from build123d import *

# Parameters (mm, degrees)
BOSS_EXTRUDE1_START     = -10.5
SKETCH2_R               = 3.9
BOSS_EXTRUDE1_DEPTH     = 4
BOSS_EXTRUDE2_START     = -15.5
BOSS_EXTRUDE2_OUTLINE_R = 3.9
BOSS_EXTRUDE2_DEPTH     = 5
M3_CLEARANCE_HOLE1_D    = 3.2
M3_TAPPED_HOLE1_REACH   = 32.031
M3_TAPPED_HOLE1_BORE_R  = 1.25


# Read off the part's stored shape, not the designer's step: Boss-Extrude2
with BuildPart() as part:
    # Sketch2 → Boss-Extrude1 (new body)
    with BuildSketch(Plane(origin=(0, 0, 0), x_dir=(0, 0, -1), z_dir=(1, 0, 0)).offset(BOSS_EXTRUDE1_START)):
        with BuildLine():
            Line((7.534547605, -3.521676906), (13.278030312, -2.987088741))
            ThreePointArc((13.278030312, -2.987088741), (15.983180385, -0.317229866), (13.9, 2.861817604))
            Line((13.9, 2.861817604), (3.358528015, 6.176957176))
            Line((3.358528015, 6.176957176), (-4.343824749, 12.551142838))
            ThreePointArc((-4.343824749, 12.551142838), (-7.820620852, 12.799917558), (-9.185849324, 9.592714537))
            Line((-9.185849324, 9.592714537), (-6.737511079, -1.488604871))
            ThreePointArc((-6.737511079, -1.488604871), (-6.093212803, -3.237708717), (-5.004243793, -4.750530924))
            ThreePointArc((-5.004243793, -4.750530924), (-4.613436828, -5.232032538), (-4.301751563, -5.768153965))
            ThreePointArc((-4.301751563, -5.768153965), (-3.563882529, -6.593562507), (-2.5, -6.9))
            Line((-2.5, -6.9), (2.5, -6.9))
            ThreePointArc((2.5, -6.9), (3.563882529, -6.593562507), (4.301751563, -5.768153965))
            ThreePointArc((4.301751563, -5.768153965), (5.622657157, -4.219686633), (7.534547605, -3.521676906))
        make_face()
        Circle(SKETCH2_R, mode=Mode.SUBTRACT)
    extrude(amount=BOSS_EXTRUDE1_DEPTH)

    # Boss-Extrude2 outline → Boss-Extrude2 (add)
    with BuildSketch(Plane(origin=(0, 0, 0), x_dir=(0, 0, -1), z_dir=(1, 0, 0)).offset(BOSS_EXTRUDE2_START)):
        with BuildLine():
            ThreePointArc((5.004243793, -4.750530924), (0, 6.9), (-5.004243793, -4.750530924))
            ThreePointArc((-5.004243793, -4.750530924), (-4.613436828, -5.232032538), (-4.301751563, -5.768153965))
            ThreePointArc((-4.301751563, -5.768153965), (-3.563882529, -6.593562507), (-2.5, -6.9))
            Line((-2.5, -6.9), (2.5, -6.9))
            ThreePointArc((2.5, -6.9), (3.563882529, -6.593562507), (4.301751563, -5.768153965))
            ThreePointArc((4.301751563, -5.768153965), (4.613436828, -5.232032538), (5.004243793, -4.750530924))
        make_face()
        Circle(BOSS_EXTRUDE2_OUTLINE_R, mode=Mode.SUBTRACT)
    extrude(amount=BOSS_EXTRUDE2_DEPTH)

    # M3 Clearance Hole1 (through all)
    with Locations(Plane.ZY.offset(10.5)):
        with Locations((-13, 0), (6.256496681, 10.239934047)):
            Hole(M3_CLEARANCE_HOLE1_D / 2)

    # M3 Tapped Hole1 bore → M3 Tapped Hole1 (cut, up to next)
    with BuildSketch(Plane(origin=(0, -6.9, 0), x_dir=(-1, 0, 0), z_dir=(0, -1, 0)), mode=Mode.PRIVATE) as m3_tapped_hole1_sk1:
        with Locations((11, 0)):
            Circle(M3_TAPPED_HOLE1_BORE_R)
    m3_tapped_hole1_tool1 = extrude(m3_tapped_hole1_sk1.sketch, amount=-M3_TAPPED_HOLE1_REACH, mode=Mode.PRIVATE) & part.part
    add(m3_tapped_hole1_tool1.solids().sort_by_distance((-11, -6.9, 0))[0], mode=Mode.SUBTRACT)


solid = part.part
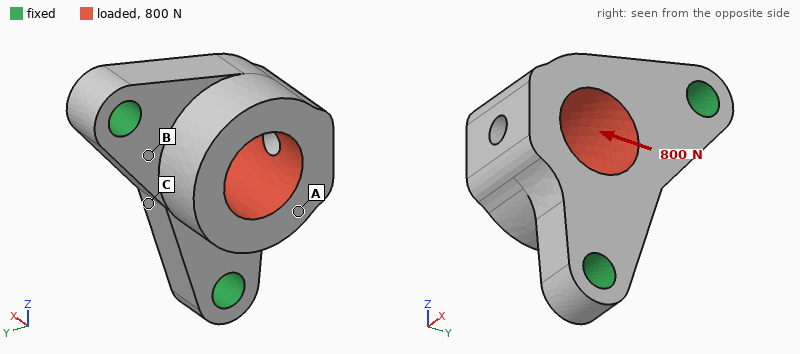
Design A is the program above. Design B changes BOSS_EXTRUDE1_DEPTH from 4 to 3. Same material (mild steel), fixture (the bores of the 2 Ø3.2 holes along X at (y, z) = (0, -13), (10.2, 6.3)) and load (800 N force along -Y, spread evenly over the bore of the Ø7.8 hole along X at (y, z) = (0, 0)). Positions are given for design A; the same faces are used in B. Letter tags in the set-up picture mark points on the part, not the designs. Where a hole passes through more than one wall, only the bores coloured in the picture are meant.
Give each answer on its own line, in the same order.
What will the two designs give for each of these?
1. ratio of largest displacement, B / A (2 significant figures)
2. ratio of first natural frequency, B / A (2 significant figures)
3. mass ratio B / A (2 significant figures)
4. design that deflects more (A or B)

1.8
0.79
0.84
B
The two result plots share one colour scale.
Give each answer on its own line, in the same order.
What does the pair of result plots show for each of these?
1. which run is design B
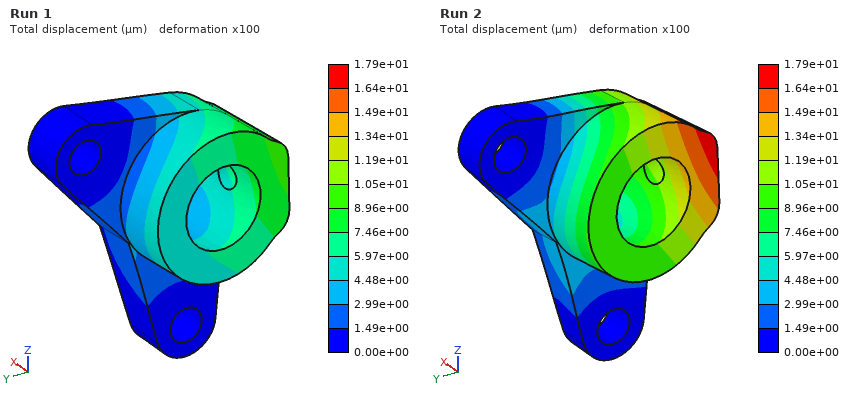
Run 2
